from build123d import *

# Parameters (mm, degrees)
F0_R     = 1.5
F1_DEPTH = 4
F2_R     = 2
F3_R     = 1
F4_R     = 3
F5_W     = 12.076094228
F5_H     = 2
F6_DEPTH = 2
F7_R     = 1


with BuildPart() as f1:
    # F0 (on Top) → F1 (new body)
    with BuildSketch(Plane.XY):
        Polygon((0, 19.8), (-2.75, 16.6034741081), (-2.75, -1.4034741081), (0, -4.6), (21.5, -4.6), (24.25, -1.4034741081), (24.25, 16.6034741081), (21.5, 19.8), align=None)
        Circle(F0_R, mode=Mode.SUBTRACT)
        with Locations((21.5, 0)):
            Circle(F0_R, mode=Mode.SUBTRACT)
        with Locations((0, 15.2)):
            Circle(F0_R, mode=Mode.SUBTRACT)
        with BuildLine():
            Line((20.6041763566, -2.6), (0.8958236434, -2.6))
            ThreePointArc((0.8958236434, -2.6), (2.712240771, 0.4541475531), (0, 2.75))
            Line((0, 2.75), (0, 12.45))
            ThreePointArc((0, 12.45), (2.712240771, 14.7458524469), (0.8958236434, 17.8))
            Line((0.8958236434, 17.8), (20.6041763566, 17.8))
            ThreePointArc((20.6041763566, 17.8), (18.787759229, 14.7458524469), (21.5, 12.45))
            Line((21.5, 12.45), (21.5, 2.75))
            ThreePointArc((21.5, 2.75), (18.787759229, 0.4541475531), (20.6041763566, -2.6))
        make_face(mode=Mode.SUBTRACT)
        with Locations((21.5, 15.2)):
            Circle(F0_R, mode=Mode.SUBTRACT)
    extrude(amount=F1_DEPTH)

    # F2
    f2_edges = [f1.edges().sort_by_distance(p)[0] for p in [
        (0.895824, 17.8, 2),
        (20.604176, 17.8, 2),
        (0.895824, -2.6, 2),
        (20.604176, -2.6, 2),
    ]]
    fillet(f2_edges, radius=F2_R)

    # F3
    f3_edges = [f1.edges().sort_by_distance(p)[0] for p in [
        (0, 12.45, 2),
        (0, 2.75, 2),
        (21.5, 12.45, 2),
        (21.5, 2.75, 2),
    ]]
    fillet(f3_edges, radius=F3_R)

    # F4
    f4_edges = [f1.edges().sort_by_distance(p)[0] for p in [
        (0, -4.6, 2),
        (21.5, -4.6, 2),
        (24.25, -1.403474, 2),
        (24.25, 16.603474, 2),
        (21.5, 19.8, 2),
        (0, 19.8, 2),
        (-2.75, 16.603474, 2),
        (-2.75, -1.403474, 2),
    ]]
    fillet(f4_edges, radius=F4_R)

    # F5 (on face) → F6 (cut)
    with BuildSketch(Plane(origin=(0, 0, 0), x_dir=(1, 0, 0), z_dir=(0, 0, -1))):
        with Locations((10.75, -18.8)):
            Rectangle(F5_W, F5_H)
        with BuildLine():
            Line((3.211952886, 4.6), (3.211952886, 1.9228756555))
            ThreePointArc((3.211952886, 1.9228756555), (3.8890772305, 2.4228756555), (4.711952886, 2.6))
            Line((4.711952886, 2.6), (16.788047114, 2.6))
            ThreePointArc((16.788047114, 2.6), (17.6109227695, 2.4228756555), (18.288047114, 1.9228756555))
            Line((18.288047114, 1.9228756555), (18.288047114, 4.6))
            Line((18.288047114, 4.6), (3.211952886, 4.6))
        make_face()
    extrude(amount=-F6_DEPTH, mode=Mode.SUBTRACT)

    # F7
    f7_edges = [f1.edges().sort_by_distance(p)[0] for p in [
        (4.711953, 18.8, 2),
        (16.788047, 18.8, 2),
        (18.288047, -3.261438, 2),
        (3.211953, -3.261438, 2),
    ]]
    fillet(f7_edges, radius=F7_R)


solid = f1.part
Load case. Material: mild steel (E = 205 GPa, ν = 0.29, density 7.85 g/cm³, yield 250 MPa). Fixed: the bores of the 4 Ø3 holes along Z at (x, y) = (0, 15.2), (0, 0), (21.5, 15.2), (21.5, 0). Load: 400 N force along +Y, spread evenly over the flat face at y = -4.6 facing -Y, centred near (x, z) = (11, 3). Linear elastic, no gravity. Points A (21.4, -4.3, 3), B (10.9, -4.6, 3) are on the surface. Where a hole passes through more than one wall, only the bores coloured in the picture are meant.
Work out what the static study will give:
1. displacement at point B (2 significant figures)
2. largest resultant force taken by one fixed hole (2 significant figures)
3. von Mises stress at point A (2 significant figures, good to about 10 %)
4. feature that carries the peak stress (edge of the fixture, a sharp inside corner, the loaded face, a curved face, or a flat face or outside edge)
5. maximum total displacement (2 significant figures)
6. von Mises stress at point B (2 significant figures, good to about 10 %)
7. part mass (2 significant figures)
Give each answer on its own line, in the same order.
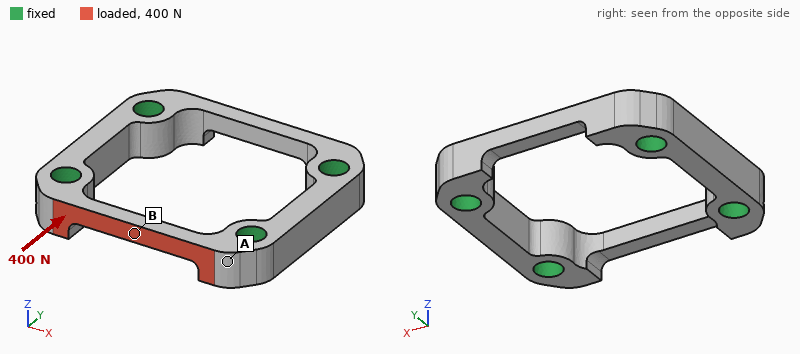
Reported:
13 µm
220 N
25 MPa
a curved face
13 µm
160 MPa
6.3 g
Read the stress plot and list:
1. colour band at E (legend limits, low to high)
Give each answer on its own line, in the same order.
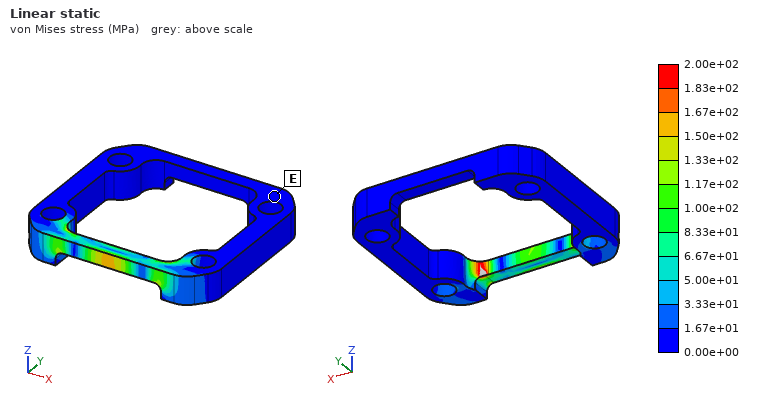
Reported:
0.00e+00 to 1.67e+01 MPa
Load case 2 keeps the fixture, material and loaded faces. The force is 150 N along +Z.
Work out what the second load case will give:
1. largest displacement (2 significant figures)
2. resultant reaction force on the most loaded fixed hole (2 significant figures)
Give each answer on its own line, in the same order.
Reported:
7.0 µm
77 N
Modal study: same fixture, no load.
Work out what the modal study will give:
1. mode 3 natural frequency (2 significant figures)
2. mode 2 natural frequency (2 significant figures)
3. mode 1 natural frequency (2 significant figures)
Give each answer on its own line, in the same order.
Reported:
39 kHz
37 kHz
35 kHz
